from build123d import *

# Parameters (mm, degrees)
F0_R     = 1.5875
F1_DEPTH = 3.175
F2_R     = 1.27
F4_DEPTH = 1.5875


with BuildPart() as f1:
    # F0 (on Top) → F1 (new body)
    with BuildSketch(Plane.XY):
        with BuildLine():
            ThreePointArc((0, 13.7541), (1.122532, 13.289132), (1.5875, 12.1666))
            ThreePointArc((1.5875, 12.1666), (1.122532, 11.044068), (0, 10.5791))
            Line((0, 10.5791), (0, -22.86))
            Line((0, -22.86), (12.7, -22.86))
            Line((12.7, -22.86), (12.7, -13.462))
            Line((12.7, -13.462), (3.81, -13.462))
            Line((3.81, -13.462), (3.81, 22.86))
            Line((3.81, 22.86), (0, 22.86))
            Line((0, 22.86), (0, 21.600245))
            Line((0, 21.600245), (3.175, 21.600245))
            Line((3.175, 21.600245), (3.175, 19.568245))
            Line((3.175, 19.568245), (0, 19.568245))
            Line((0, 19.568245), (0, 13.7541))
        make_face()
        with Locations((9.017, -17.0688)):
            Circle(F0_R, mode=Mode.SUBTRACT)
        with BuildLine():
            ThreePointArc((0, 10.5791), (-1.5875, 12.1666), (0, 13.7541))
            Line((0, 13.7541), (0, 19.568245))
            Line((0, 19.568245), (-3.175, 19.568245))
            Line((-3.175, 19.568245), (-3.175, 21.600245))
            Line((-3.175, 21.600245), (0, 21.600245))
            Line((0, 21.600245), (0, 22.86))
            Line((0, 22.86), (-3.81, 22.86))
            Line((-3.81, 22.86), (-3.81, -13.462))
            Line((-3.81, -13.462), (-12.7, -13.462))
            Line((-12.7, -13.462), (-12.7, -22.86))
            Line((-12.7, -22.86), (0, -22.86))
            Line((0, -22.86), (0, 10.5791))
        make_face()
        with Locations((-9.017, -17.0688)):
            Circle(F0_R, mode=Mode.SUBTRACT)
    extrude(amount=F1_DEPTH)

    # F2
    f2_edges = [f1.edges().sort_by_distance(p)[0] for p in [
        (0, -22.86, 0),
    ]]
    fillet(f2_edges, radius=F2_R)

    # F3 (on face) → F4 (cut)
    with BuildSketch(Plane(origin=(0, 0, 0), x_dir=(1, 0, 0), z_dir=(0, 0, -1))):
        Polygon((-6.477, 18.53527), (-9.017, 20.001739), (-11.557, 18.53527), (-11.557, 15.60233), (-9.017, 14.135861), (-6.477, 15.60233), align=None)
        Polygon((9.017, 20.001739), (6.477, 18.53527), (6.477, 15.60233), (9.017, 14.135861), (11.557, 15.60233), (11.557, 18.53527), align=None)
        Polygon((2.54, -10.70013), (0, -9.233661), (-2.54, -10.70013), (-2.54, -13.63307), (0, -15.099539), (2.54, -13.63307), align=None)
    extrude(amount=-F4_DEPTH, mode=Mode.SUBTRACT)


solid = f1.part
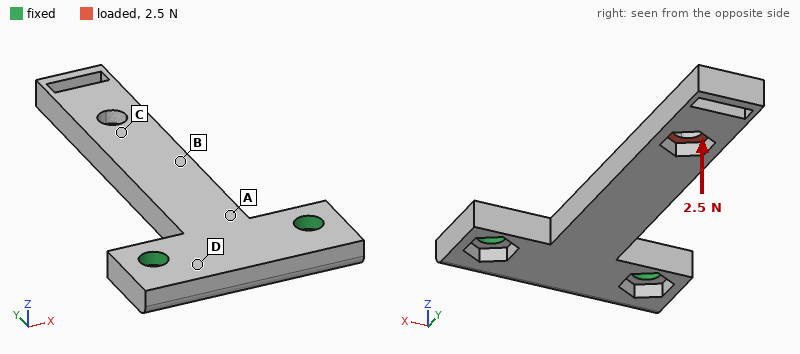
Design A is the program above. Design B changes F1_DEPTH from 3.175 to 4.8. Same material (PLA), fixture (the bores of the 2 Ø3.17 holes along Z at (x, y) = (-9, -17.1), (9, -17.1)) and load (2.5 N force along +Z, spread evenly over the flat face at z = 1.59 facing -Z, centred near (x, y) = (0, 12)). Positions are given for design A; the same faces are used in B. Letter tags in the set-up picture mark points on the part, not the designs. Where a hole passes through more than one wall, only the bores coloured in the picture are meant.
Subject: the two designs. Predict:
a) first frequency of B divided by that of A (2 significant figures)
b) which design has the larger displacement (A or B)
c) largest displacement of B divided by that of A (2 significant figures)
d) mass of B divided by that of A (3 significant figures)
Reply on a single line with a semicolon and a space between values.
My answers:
1.5; A; 0.30; 1.54
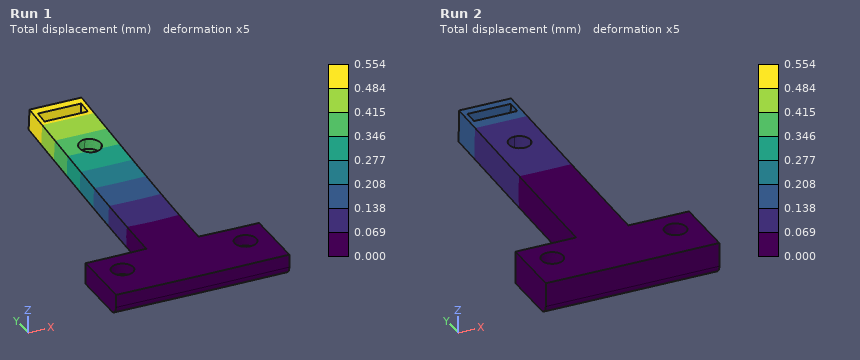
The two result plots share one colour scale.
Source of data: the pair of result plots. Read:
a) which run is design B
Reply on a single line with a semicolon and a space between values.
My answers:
Run 2
